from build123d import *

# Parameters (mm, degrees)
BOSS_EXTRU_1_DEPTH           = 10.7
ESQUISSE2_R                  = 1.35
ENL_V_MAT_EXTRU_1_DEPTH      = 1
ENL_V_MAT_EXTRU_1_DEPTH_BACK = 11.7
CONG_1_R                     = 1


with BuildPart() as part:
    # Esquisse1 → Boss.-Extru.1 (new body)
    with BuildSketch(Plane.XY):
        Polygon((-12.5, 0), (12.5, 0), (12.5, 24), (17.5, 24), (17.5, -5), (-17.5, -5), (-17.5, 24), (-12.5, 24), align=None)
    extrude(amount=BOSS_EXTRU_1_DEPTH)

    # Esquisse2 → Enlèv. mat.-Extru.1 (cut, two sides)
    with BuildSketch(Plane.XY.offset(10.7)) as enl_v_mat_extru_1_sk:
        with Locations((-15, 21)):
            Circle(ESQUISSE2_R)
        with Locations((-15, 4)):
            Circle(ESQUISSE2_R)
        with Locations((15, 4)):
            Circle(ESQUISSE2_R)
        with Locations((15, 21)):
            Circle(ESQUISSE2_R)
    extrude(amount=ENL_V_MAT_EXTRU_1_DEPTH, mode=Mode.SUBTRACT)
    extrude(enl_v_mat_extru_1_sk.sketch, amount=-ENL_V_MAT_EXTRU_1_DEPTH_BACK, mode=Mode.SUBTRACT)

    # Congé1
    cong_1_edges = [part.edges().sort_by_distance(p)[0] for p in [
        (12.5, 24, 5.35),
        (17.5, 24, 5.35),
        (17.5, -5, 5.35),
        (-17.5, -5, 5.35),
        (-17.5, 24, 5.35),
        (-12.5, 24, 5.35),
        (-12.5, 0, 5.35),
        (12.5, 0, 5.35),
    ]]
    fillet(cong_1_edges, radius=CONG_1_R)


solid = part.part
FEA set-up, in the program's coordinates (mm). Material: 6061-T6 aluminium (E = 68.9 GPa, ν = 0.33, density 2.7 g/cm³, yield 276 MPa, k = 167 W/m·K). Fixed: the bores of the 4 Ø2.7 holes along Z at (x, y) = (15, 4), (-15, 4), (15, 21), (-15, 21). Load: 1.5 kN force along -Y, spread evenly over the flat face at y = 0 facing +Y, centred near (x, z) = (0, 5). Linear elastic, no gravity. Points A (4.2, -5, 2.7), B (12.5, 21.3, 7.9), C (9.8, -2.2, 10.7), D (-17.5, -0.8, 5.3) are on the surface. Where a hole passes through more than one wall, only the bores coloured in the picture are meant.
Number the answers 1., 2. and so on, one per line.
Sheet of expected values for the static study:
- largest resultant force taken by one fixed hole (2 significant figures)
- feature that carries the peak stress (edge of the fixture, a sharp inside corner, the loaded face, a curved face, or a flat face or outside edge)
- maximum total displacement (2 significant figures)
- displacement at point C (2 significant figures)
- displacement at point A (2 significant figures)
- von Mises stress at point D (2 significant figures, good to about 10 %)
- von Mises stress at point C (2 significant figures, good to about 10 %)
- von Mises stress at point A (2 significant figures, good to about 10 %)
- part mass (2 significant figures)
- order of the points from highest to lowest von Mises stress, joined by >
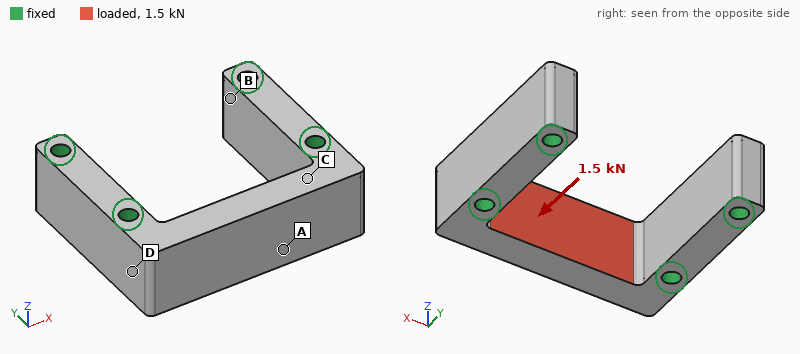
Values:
1. 990 N
2. a curved face
3. 25 µm
4. 9.0 µm
5. 20 µm
6. 26 MPa
7. 41 MPa
8. 55 MPa
9. 11 g
10. A > C > D > B
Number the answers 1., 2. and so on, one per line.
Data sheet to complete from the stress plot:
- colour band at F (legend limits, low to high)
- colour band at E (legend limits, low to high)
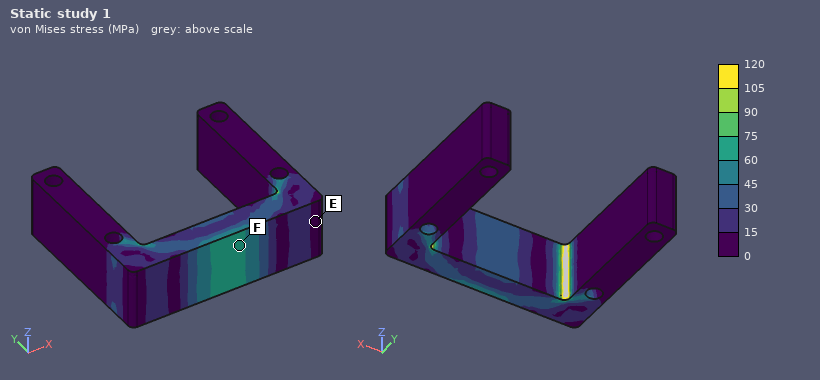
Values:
1. 60 to 75 MPa
2. 0 to 15 MPa
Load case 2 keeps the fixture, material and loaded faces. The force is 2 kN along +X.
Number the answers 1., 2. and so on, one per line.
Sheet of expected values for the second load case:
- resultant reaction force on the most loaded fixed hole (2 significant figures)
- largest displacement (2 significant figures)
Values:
1. 1.0 kN
2. 13 µm
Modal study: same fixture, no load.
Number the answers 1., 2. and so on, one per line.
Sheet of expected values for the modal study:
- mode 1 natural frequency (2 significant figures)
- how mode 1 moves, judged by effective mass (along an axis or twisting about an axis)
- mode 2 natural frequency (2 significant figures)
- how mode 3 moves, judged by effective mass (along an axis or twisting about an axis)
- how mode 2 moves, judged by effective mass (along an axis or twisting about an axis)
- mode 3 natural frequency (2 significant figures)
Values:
1. 24 kHz
2. along Y
3. 26 kHz
4. along X
5. along Z
6. 31 kHz
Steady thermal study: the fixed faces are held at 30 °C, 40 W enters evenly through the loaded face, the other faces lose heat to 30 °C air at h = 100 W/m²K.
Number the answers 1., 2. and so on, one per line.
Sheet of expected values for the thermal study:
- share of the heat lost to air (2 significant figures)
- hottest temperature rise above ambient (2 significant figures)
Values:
1. 3.7 %
2. 28 K
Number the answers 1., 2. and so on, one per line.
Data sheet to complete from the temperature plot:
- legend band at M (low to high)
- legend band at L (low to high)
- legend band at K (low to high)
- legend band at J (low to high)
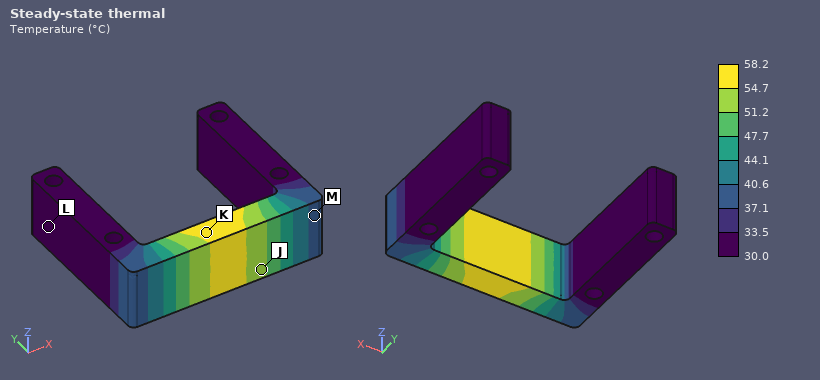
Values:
1. 37.1 to 40.6 °C
2. 30.0 to 33.5 °C
3. 54.7 to 58.2 °C
4. 51.2 to 54.7 °C
